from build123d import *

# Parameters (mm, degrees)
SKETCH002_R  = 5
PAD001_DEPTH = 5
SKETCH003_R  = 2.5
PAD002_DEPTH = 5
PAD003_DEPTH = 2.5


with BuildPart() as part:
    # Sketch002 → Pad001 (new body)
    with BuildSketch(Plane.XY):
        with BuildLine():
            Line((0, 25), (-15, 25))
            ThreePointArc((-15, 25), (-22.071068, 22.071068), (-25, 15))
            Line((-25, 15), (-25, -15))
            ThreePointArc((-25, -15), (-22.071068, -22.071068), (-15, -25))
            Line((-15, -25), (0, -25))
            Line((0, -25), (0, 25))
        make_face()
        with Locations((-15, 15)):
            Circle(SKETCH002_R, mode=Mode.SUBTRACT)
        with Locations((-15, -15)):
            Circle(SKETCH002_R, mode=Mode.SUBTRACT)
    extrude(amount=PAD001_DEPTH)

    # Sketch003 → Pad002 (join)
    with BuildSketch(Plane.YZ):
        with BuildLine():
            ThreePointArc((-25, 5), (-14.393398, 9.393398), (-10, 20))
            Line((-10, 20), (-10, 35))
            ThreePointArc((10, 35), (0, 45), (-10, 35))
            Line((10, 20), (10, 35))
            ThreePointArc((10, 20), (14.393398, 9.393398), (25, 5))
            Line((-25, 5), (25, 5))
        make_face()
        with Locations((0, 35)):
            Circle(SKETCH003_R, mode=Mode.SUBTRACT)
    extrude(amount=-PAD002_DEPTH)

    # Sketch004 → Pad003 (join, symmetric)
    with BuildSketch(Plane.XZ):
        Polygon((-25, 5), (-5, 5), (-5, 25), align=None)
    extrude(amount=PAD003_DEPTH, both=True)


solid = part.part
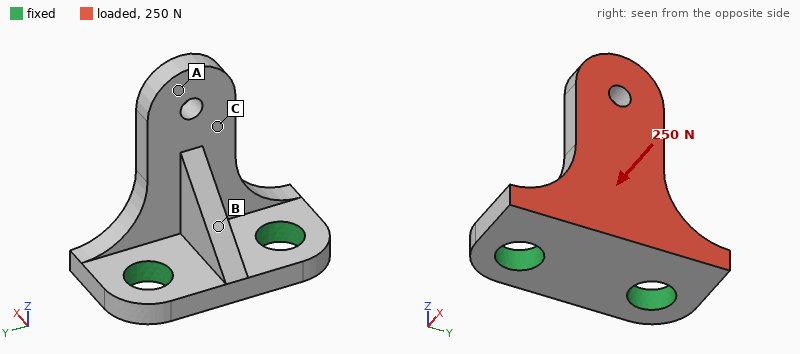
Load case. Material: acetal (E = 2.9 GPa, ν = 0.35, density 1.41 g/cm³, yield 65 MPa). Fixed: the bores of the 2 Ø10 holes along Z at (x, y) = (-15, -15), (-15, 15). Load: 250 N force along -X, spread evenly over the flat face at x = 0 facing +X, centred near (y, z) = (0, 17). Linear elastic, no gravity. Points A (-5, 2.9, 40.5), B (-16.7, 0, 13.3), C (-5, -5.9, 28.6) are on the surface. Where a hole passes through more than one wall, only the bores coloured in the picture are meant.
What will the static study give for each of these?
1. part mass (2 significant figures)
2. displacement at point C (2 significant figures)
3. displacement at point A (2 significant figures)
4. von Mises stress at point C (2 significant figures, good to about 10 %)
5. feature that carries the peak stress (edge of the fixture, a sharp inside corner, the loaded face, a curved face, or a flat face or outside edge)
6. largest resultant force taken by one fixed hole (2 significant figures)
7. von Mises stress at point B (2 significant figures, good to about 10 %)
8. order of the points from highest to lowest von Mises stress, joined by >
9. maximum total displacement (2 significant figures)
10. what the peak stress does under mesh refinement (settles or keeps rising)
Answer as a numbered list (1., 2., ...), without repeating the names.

1. 15 g
2. 0.34 mm
3. 0.64 mm
4. 4.9 MPa
5. edge of the fixture
6. 130 N
7. 8.0 MPa
8. B > C > A
9. 0.77 mm
10. keeps rising
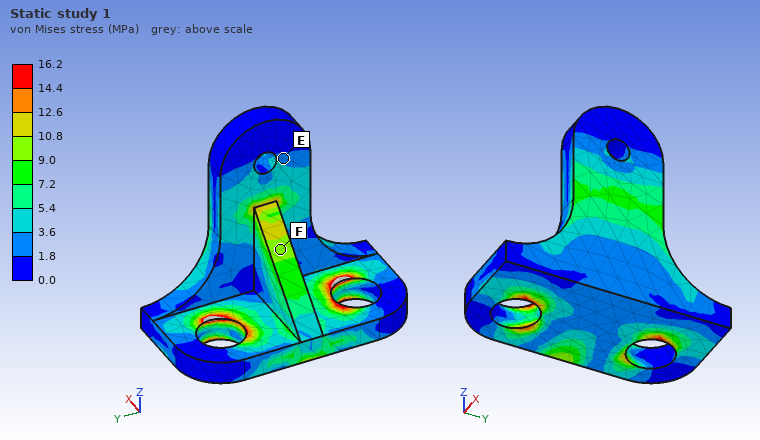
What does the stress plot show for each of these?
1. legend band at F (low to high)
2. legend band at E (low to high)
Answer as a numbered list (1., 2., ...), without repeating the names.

1. 9.0 to 10.8 MPa
2. 1.8 to 3.6 MPa
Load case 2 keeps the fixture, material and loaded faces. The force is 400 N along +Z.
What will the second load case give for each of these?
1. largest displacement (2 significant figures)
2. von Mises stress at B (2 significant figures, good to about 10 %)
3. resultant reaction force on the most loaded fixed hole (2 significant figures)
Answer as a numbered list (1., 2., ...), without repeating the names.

1. 0.58 mm
2. 4.8 MPa
3. 210 N
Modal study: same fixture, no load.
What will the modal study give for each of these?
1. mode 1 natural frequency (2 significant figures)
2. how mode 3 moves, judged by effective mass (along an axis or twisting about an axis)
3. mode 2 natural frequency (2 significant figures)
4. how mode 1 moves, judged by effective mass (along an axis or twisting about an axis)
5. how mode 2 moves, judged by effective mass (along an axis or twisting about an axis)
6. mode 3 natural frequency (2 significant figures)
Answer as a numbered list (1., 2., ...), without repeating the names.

1. 1300 Hz
2. along Z
3. 2400 Hz
4. along X
5. along Y
6. 3500 Hz
